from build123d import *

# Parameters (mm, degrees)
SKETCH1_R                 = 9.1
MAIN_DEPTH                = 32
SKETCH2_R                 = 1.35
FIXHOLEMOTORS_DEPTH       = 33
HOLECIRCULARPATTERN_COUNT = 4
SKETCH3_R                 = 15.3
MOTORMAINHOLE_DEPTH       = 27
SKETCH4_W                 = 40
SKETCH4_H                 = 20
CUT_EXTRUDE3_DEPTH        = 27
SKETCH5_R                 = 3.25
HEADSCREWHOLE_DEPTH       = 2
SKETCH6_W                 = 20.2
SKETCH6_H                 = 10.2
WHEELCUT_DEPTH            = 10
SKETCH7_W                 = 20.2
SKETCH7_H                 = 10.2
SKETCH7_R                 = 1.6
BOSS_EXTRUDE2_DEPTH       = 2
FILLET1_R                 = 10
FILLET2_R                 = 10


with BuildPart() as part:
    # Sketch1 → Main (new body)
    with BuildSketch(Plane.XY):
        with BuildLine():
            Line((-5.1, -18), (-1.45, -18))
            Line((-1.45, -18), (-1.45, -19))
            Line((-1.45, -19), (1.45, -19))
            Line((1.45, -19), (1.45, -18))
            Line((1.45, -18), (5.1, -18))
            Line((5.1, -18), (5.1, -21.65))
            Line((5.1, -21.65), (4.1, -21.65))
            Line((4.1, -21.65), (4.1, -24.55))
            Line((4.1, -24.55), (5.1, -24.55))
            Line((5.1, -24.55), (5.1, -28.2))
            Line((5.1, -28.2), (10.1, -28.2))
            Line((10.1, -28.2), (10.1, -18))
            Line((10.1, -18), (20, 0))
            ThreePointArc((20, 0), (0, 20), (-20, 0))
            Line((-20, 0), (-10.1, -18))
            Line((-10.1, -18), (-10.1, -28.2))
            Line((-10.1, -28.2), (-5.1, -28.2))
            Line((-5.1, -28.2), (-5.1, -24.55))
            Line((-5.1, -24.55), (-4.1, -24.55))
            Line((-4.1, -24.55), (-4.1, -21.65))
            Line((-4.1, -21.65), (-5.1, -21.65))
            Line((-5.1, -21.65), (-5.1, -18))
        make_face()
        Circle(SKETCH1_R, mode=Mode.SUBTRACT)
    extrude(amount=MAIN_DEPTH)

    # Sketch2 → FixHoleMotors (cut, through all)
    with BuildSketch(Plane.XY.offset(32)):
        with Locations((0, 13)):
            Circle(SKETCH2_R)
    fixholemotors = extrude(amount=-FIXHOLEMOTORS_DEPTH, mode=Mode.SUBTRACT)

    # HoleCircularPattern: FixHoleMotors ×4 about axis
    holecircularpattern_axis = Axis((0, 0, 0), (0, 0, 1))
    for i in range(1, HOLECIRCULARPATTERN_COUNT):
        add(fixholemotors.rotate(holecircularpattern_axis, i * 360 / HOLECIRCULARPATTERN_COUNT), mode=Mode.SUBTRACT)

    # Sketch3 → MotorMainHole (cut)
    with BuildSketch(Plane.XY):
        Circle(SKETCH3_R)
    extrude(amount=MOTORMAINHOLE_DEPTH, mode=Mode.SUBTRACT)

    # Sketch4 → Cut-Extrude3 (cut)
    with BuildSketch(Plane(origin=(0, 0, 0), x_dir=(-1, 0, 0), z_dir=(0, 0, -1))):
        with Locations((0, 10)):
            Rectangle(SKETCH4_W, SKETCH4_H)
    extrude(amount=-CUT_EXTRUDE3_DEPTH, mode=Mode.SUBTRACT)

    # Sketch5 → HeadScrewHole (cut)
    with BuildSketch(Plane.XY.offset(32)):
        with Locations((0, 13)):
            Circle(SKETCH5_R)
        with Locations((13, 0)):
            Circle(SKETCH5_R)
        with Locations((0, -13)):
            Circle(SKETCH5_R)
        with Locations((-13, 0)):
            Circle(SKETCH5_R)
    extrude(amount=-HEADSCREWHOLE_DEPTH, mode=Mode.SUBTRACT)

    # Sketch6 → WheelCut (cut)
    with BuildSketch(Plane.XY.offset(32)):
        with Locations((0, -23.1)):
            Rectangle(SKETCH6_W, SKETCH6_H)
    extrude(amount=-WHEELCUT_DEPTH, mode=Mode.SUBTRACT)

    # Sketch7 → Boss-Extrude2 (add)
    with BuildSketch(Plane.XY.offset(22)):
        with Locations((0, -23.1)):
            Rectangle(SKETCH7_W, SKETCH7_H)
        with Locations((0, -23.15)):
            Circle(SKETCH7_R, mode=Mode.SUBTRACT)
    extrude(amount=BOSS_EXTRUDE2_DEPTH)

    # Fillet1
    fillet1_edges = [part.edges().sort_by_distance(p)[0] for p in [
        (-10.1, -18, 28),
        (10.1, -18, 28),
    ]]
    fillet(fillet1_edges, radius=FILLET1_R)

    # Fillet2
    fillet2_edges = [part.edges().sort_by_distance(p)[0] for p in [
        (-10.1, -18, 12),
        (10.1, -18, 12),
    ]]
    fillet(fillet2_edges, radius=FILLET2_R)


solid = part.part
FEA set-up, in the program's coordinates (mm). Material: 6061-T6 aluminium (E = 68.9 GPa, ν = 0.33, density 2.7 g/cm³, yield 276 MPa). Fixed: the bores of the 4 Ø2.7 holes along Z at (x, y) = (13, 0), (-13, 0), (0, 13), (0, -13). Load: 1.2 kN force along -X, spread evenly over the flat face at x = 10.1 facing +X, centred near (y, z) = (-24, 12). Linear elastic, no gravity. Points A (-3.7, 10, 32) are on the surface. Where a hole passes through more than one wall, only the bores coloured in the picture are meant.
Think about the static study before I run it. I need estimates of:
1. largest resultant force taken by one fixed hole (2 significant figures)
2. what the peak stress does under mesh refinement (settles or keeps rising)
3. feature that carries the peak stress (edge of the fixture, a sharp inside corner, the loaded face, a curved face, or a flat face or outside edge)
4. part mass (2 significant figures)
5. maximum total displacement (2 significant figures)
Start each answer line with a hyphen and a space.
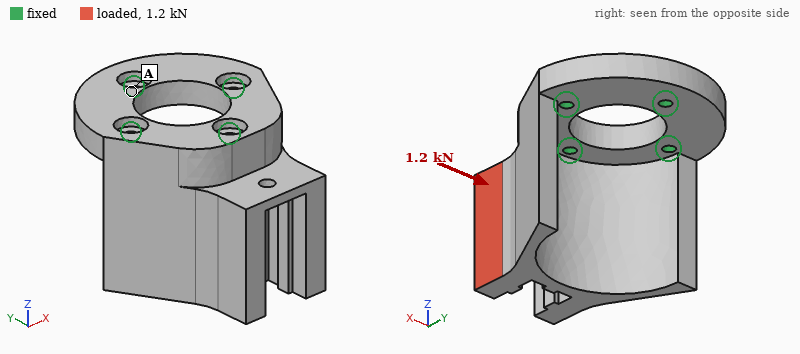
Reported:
- 940 N
- keeps rising
- edge of the fixture
- 32 g
- 80 µm
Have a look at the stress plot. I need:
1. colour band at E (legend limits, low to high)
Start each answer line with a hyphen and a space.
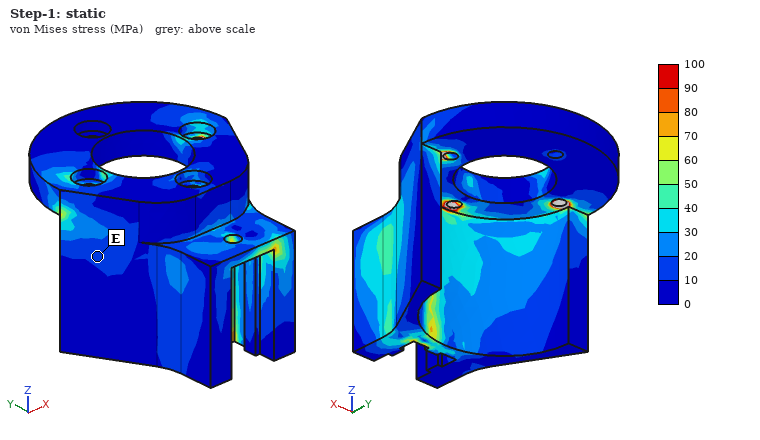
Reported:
- 10 to 20 MPa
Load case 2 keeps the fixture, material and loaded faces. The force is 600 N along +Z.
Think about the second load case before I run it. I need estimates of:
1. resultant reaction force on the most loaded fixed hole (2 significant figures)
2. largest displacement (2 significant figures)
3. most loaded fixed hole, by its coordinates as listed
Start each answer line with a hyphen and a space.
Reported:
- 980 N
- 63 µm
- (0, -13)
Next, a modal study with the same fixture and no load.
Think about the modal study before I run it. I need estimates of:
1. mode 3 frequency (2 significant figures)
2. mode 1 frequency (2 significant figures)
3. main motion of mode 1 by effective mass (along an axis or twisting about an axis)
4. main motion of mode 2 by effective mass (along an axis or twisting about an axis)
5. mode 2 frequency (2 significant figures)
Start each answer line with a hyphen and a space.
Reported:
- 8700 Hz
- 4400 Hz
- along X
- along Y
- 5500 Hz
